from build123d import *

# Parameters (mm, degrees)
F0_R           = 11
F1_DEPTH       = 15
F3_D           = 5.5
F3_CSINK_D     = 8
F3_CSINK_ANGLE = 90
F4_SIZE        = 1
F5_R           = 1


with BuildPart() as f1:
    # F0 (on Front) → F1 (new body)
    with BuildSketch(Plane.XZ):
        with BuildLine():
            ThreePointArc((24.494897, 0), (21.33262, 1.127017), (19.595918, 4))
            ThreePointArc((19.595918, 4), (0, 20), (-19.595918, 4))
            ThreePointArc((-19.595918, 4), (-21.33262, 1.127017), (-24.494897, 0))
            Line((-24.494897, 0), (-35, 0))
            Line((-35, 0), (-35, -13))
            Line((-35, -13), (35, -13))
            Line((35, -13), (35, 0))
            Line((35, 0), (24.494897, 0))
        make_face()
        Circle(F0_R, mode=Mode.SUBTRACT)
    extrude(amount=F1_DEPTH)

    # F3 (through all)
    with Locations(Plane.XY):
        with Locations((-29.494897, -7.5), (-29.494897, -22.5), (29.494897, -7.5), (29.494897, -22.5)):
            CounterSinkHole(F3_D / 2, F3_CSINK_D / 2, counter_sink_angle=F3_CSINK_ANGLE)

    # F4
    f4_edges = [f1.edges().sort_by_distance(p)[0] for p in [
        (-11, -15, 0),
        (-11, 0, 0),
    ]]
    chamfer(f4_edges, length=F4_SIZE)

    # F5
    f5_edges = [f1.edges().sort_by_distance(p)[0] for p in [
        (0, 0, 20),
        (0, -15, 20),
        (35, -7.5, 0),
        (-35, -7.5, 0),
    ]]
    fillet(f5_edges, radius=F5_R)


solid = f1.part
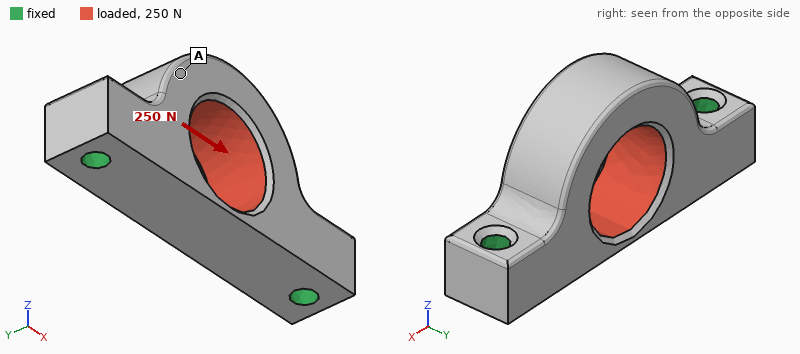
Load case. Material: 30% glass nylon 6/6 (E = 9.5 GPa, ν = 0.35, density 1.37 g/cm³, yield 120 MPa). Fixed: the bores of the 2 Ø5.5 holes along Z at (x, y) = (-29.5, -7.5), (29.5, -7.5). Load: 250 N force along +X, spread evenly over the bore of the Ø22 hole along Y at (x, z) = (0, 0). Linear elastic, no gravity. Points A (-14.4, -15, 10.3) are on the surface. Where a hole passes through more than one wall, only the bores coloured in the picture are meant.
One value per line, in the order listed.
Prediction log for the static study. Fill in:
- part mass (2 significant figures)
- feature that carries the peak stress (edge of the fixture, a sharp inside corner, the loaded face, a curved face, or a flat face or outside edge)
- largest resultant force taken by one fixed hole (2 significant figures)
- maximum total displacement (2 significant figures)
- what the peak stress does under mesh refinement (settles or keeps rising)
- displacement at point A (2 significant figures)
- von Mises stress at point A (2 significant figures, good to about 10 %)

23 g
edge of the fixture
130 N
4.4 µm
keeps rising
4.0 µm
0.34 MPa
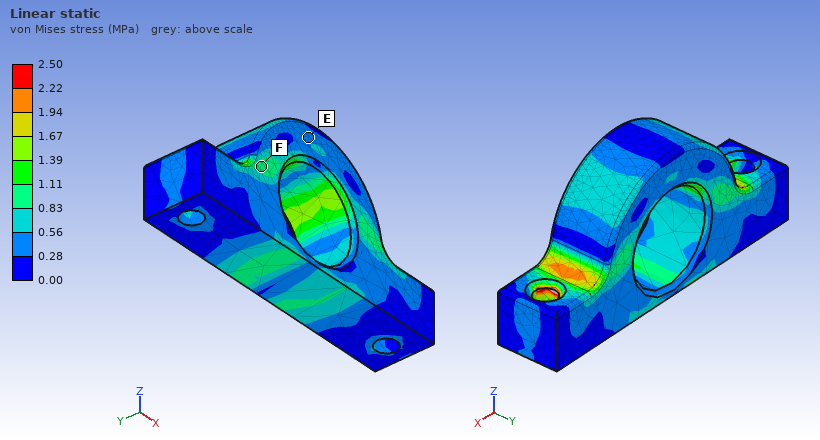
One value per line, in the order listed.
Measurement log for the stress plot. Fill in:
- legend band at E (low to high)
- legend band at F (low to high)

0.28 to 0.56 MPa
0.83 to 1.11 MPa
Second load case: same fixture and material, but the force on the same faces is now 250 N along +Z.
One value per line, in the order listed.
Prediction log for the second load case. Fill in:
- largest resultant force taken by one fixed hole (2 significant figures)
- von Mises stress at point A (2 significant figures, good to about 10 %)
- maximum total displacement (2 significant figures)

130 N
0.79 MPa
9.8 µm
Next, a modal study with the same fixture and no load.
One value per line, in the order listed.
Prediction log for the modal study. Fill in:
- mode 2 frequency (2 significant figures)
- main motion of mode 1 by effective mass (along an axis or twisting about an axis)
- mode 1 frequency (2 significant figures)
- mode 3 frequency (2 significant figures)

9000 Hz
along Y
4100 Hz
9200 Hz
